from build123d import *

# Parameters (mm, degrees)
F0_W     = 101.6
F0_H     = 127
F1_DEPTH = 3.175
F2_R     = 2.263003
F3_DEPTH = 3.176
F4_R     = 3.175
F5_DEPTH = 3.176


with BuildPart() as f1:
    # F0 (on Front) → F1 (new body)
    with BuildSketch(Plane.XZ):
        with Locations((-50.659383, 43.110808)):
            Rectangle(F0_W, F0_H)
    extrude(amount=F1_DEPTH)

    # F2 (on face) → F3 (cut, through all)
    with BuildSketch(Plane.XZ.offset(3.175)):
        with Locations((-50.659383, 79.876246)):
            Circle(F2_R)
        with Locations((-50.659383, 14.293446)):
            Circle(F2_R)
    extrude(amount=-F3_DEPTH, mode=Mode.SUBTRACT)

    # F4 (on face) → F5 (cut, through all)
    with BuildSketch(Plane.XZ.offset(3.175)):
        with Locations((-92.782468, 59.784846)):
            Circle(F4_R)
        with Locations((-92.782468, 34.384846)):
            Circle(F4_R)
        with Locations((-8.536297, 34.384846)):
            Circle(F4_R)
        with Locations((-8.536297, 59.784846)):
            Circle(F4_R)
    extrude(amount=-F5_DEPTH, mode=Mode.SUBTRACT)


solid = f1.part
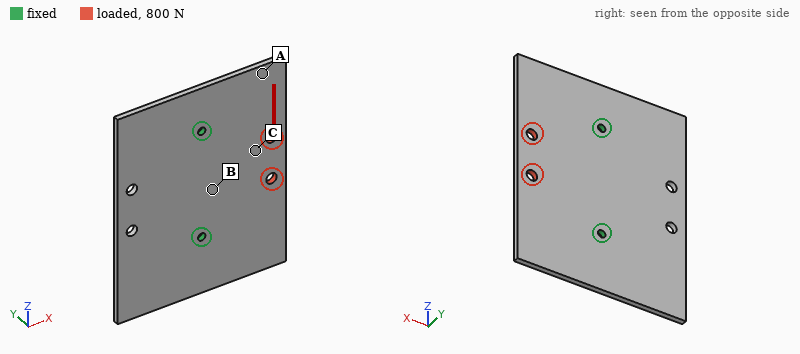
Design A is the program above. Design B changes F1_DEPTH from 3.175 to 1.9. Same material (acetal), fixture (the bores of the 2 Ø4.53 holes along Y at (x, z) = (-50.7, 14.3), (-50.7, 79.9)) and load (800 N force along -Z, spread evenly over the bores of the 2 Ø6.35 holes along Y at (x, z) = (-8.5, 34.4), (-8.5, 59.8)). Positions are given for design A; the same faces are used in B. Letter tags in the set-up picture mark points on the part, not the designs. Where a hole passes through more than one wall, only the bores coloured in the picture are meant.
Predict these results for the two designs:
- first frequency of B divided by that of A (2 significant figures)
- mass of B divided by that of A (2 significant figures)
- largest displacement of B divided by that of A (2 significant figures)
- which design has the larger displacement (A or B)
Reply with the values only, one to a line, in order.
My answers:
0.63
0.60
1.7
B
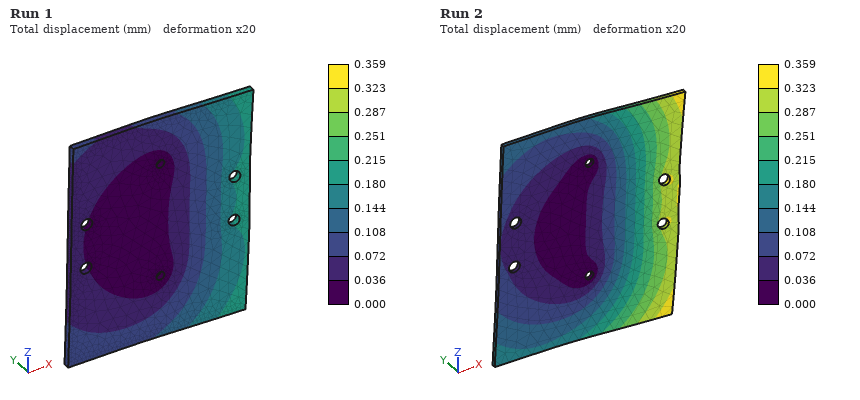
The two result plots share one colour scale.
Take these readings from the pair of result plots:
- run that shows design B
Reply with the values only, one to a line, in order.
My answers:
Run 2
